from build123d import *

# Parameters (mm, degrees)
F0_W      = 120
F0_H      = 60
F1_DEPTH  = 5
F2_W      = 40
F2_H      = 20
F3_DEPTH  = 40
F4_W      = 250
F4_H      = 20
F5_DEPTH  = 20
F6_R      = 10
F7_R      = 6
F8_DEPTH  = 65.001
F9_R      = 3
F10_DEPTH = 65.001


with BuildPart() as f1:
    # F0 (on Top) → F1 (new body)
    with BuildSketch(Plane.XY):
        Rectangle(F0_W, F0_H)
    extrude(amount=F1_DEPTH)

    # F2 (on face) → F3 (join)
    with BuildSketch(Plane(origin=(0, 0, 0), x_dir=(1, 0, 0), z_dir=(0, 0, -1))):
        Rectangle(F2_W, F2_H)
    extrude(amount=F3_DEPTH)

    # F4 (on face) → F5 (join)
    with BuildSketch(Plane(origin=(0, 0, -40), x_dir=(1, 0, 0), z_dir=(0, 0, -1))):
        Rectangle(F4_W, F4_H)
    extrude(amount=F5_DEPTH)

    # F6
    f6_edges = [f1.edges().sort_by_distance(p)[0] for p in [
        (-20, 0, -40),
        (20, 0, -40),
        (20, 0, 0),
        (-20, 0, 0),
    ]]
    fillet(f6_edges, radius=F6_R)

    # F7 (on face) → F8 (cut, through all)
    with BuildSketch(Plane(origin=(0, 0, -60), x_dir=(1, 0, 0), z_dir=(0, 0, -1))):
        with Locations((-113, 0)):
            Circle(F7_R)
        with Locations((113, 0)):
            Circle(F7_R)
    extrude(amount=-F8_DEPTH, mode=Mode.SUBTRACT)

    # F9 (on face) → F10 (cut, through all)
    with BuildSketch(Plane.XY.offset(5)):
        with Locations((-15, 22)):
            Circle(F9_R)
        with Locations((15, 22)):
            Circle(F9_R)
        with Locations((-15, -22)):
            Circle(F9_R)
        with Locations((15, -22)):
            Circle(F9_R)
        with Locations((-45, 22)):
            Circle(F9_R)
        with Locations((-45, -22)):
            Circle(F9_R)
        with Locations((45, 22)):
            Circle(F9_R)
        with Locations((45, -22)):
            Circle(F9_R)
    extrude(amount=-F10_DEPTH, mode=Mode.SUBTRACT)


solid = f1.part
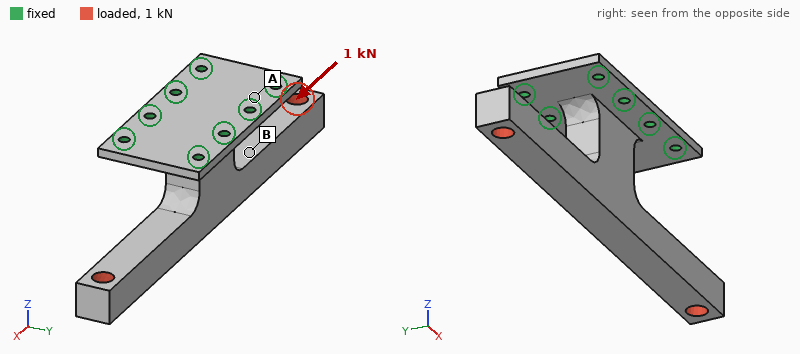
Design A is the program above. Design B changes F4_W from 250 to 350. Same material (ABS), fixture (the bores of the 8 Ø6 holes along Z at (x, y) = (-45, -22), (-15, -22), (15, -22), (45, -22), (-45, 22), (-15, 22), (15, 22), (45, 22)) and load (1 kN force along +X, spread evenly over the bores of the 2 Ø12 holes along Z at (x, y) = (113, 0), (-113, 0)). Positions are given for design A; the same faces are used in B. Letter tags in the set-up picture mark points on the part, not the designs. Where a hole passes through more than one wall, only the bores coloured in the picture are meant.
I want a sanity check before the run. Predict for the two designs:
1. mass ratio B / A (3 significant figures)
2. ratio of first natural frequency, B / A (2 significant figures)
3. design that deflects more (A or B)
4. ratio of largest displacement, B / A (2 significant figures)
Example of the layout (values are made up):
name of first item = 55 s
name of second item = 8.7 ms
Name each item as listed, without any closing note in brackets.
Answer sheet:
mass ratio B / A = 1.24
ratio of first natural frequency, B / A = 0.53
design that deflects more = B
ratio of largest displacement, B / A = 1.3
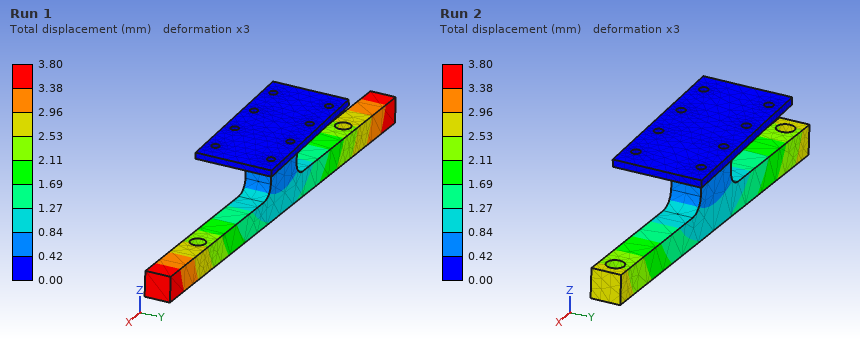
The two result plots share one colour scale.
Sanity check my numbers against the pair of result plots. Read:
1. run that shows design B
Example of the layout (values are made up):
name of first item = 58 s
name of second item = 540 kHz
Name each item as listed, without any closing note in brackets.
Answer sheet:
run that shows design B = Run 1
